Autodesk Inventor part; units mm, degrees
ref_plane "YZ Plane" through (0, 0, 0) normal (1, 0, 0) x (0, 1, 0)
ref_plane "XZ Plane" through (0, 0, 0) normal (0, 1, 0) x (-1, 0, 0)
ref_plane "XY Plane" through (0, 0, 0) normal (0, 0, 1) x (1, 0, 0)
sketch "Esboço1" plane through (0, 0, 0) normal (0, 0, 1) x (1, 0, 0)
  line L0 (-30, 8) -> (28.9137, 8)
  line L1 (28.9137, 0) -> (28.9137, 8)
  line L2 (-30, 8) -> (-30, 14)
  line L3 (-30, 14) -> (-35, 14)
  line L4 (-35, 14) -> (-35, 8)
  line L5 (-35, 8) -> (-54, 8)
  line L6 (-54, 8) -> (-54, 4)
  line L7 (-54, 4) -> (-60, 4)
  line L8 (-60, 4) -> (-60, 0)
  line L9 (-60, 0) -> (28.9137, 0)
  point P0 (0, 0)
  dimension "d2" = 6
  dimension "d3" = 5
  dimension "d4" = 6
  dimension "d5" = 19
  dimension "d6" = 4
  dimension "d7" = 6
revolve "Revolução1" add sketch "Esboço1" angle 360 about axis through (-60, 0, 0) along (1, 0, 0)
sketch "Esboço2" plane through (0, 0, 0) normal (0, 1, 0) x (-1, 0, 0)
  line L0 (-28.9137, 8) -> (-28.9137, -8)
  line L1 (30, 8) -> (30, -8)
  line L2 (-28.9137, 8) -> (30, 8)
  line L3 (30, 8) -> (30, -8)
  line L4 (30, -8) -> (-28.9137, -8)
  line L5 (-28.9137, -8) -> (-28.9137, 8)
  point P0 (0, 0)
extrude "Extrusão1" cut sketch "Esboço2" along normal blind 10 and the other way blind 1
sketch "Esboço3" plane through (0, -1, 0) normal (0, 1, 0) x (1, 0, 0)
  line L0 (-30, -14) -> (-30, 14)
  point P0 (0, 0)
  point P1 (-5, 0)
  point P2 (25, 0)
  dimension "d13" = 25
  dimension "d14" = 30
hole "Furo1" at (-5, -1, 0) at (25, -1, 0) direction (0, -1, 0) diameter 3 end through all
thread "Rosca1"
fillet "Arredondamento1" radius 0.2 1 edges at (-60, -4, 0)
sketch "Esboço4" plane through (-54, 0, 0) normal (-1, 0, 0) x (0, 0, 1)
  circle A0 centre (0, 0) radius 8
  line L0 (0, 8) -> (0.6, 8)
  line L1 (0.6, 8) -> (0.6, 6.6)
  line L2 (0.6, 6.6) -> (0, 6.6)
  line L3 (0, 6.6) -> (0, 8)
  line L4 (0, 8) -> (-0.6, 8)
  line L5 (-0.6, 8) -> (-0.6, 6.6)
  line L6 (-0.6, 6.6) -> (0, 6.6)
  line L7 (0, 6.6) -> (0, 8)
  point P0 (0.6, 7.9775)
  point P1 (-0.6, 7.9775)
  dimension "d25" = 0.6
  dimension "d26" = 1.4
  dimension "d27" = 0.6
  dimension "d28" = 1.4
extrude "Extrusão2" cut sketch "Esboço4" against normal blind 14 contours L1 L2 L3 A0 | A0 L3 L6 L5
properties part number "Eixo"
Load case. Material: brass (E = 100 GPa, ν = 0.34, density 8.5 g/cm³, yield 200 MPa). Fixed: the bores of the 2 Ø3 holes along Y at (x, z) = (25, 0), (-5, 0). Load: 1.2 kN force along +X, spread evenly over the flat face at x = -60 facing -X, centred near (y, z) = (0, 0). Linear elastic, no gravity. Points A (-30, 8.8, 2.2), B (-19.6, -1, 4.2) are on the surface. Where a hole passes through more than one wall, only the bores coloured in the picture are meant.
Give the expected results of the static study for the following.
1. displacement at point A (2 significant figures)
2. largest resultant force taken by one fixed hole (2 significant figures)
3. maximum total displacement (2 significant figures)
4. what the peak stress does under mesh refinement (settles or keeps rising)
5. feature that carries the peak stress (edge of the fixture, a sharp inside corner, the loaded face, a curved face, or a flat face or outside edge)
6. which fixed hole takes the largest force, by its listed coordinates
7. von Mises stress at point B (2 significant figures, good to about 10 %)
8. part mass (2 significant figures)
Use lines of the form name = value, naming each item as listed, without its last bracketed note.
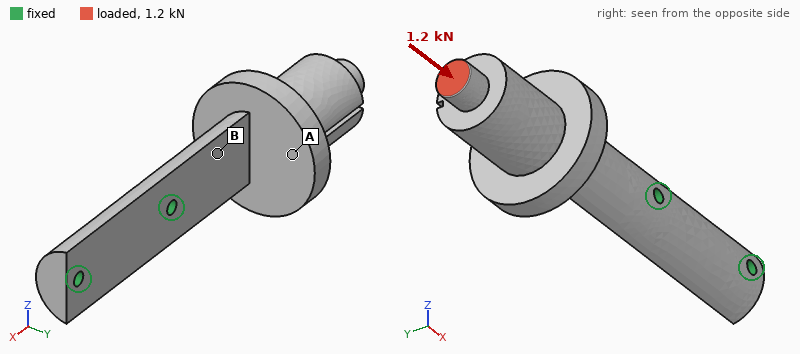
displacement at point A = 0.081 mm
largest resultant force taken by one fixed hole = 1.1 kN
maximum total displacement = 0.19 mm
what the peak stress does under mesh refinement = keeps rising
feature that carries the peak stress = edge of the fixture
which fixed hole takes the largest force, by its listed coordinates = (-5, 0)
von Mises stress at point B = 63 MPa
part mass = 100 g
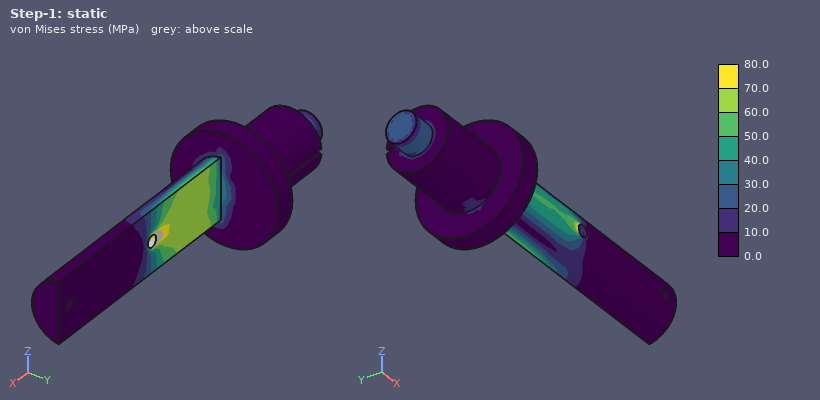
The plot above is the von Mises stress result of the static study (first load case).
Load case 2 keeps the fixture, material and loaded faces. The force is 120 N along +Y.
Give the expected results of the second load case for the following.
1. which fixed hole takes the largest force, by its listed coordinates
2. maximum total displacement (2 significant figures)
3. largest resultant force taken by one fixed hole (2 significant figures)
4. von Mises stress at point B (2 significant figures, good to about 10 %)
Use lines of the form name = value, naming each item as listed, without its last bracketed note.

which fixed hole takes the largest force, by its listed coordinates = (-5, 0)
maximum total displacement = 0.21 mm
largest resultant force taken by one fixed hole = 170 N
von Mises stress at point B = 49 MPa
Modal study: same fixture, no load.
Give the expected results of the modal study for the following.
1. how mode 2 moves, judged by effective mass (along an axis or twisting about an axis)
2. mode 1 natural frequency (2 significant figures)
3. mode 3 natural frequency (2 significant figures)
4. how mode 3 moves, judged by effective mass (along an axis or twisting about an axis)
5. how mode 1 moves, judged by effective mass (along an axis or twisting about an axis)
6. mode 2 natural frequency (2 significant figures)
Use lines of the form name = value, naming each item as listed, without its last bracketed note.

how mode 2 moves, judged by effective mass = along Z
mode 1 natural frequency = 840 Hz
mode 3 natural frequency = 2900 Hz
how mode 3 moves, judged by effective mass = twisting about X
how mode 1 moves, judged by effective mass = along Y
mode 2 natural frequency = 1300 Hz
